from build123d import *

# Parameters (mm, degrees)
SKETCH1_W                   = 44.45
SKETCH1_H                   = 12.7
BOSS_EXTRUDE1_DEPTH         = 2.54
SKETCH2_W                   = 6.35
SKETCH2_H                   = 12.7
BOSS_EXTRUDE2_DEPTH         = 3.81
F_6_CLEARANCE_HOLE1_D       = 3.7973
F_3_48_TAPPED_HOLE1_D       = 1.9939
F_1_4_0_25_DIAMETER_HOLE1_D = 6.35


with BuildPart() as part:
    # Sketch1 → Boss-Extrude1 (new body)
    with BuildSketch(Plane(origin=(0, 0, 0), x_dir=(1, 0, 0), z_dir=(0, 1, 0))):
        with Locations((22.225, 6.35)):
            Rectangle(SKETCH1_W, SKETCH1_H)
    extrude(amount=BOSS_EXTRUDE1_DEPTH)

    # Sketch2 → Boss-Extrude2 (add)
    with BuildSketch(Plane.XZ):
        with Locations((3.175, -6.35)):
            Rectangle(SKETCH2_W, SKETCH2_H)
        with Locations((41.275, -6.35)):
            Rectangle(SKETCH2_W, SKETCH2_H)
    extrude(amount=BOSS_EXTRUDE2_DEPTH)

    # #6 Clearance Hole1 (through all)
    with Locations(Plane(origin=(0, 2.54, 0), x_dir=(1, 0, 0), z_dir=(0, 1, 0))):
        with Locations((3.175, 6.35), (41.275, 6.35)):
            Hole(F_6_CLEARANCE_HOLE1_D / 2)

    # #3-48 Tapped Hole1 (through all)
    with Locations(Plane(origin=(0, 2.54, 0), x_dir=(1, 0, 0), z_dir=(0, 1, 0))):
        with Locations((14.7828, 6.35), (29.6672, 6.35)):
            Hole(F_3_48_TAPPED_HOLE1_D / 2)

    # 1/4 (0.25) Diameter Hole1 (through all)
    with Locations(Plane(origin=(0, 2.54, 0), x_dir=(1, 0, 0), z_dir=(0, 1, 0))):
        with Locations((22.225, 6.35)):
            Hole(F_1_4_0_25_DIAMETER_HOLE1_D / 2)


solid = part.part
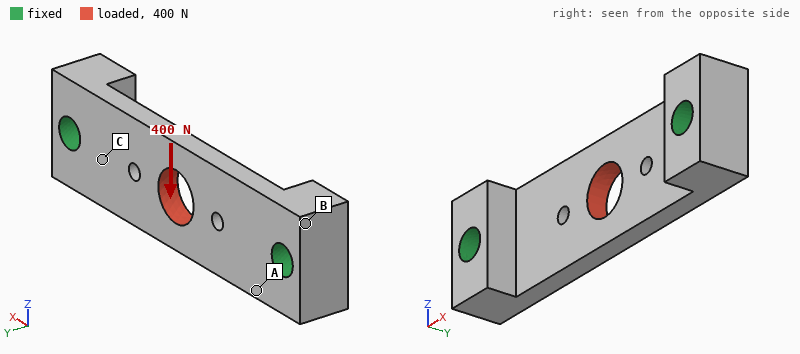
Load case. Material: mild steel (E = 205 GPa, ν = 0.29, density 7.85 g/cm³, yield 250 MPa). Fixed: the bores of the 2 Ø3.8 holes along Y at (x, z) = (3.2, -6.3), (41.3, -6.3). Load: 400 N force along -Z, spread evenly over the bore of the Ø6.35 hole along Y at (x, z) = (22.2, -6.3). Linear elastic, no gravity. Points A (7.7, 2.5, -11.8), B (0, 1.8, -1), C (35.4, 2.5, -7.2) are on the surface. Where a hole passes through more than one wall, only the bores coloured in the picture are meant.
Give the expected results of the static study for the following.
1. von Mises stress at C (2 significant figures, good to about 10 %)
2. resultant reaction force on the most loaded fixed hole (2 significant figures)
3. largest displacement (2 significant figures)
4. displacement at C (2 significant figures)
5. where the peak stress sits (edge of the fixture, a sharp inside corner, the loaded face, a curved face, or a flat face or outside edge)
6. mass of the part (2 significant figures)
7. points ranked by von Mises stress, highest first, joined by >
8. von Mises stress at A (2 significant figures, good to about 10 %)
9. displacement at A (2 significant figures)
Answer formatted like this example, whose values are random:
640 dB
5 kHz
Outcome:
15 MPa
200 N
3.5 µm
0.88 µm
edge of the fixture
14 g
C > A > B
8.0 MPa
0.95 µm
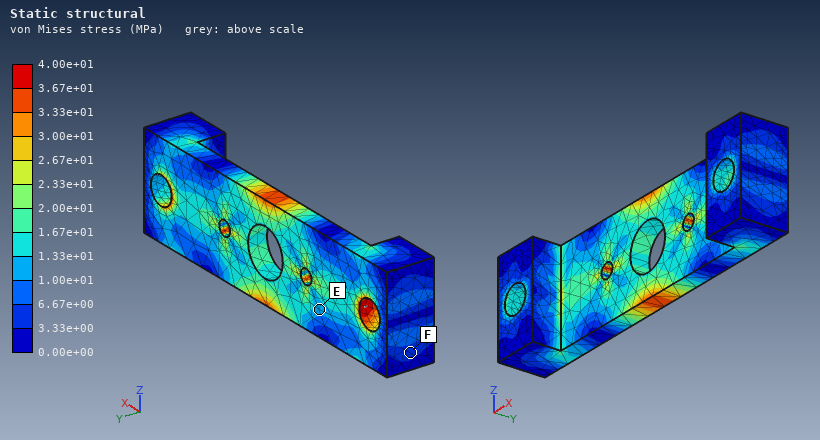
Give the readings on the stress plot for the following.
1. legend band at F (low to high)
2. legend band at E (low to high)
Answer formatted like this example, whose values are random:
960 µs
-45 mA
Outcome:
3.33e+00 to 6.67e+00 MPa
1.00e+01 to 1.33e+01 MPa
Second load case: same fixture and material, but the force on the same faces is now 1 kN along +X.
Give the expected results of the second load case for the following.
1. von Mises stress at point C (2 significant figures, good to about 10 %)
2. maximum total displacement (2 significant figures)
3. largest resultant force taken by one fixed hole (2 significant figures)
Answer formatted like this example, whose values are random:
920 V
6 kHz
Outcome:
17 MPa
1.6 µm
500 N
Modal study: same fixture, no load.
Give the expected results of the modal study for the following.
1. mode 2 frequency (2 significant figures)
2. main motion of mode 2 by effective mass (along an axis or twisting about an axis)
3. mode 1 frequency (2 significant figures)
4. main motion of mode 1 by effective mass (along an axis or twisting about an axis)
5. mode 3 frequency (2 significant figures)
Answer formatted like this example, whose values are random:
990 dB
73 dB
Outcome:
20 kHz
twisting about X
11 kHz
along Y
28 kHz
